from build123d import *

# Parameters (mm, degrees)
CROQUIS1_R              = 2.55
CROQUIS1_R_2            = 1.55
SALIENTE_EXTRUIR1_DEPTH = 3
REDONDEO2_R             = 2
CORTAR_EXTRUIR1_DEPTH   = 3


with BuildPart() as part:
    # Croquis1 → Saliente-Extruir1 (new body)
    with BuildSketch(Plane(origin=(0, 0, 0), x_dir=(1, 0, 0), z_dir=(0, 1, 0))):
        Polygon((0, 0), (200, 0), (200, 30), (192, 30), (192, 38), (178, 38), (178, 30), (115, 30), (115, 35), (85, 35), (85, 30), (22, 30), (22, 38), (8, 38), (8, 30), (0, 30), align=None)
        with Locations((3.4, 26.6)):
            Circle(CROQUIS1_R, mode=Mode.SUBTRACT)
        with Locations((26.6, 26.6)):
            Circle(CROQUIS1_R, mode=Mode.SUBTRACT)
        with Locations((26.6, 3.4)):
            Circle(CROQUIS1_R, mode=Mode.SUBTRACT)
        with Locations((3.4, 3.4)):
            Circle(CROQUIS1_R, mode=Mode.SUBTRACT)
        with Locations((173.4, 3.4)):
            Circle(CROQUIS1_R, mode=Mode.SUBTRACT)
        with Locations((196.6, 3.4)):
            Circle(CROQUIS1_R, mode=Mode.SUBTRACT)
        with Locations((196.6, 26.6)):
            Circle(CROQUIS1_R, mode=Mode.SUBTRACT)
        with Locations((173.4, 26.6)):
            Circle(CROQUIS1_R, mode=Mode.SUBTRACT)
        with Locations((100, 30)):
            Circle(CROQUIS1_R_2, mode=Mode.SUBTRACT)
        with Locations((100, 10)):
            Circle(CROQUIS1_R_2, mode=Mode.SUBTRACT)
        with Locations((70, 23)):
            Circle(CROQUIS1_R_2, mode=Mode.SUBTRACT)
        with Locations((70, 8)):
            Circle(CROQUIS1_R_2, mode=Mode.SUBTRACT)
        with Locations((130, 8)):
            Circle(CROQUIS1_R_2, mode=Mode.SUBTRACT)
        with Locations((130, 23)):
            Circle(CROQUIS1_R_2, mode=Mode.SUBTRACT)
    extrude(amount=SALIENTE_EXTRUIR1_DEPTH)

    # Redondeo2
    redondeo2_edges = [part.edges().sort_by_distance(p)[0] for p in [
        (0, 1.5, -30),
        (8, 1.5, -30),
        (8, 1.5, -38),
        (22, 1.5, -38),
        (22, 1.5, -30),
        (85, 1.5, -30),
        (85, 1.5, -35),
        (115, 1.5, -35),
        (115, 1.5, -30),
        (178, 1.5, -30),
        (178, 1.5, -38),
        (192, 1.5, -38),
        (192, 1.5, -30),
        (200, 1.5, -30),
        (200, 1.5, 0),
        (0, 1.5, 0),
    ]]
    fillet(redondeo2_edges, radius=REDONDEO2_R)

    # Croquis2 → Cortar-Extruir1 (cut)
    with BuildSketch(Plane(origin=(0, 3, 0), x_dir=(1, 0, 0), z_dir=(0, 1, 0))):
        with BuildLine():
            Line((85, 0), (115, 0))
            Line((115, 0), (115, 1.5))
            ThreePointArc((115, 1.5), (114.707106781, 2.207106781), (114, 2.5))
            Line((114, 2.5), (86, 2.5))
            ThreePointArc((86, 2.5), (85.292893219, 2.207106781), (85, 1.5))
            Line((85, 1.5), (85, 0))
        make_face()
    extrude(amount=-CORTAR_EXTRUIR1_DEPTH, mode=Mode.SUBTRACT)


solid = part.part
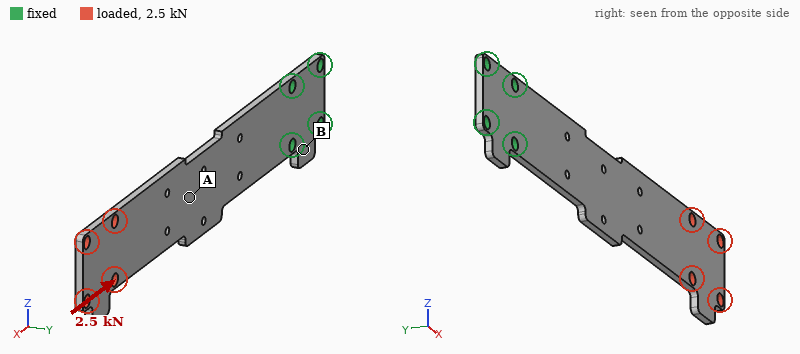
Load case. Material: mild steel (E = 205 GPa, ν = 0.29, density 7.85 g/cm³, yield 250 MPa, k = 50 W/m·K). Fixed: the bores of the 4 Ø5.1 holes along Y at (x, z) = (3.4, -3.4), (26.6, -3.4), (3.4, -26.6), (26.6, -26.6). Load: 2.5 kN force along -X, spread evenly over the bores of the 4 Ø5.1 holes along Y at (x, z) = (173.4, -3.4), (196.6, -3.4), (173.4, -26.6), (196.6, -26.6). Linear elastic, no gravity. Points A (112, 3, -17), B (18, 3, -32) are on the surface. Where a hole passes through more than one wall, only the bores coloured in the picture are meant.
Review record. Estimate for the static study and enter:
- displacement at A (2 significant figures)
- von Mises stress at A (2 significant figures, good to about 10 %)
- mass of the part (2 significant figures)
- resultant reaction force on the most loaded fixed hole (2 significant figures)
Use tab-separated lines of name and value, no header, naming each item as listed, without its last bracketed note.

displacement at A	12 µm
von Mises stress at A	28 MPa
mass of the part	140 g
resultant reaction force on the most loaded fixed hole	1.2 kN
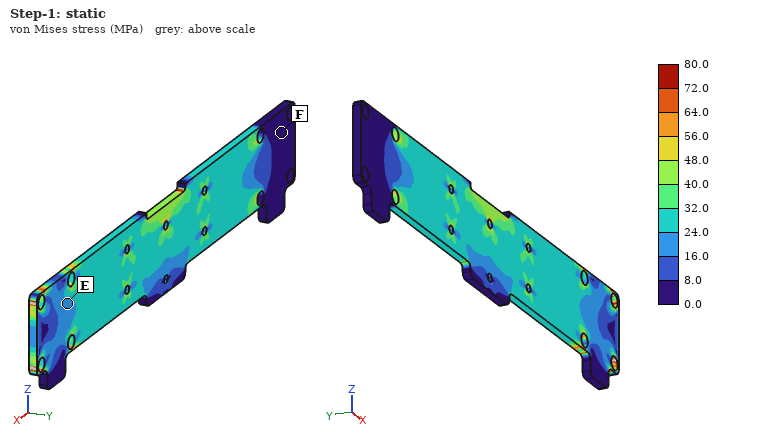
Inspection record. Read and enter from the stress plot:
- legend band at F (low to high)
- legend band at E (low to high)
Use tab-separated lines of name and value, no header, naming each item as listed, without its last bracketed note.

legend band at F	0.0 to 8.0 MPa
legend band at E	16.0 to 24.0 MPa
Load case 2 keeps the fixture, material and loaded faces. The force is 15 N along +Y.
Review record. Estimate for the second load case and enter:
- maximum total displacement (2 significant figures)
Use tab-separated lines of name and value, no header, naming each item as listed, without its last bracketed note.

maximum total displacement	1.6 mm
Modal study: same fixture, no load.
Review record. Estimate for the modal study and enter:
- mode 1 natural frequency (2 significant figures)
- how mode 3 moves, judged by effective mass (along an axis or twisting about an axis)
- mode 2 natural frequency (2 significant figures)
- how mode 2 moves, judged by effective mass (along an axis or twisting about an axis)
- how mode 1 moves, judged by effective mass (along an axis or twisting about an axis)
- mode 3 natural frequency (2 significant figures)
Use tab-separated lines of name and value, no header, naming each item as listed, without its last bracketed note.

mode 1 natural frequency	82 Hz
how mode 3 moves, judged by effective mass	along Z
mode 2 natural frequency	510 Hz
how mode 2 moves, judged by effective mass	along Y
how mode 1 moves, judged by effective mass	along Y
mode 3 natural frequency	800 Hz
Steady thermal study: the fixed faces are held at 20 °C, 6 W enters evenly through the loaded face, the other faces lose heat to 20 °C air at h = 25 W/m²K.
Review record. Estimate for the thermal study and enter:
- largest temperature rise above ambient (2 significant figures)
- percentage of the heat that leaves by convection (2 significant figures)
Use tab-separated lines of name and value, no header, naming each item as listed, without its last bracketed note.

largest temperature rise above ambient	59 K
percentage of the heat that leaves by convection	93 %
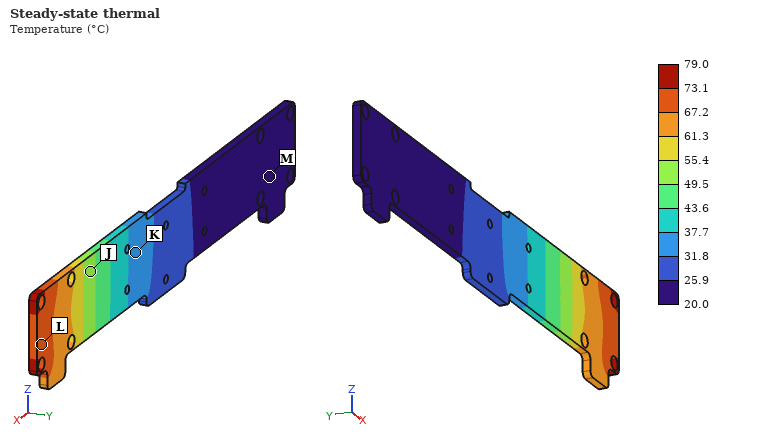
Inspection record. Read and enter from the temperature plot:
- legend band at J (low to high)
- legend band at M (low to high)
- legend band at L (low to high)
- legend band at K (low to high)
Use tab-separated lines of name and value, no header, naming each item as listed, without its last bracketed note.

legend band at J	49.5 to 55.4 °C
legend band at M	20.0 to 25.9 °C
legend band at L	67.2 to 73.1 °C
legend band at K	31.8 to 37.7 °C
